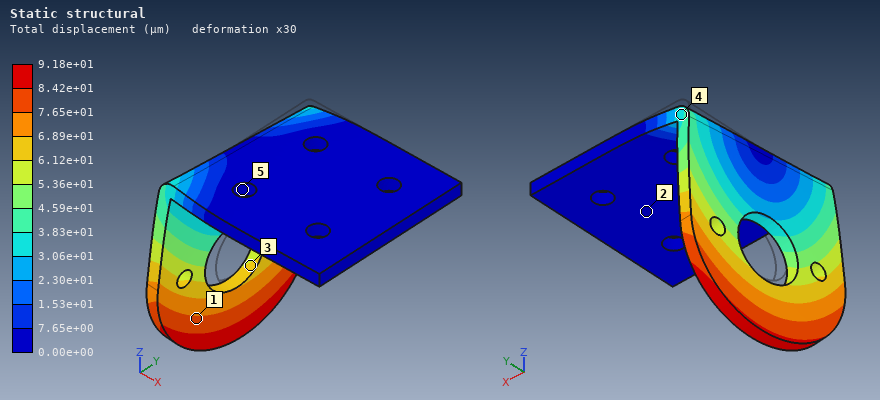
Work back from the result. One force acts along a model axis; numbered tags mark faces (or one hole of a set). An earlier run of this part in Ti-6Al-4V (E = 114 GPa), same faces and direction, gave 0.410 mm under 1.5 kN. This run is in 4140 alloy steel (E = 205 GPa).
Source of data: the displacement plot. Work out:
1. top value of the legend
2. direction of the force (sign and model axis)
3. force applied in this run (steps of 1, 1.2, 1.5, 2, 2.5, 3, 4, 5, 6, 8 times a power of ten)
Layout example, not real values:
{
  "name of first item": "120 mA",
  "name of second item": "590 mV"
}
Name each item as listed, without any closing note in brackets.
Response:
{
  "top value of the legend": "9.18e+01 µm",
  "direction of the force": "-Y",
  "force applied in this run": "600 N"
}
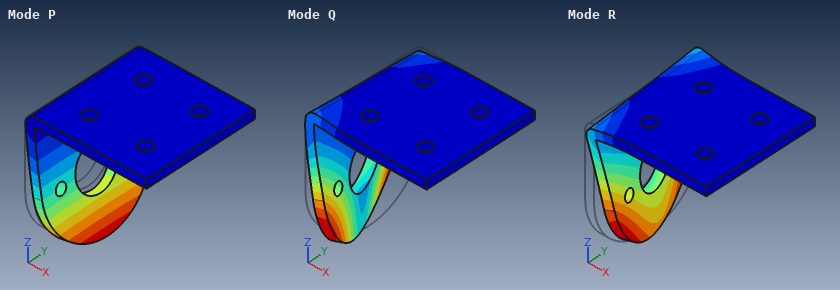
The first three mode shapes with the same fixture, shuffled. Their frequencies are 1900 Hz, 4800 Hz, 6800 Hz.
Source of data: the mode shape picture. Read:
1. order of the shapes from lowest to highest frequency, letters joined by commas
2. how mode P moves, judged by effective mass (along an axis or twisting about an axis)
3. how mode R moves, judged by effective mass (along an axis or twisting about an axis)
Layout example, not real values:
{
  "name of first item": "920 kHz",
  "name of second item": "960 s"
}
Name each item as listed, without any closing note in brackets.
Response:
{
  "order of the shapes from lowest to highest frequency, letters joined by commas": "P, R, Q",
  "how mode P moves, judged by effective mass": "along X",
  "how mode R moves, judged by effective mass": "along Y"
}
